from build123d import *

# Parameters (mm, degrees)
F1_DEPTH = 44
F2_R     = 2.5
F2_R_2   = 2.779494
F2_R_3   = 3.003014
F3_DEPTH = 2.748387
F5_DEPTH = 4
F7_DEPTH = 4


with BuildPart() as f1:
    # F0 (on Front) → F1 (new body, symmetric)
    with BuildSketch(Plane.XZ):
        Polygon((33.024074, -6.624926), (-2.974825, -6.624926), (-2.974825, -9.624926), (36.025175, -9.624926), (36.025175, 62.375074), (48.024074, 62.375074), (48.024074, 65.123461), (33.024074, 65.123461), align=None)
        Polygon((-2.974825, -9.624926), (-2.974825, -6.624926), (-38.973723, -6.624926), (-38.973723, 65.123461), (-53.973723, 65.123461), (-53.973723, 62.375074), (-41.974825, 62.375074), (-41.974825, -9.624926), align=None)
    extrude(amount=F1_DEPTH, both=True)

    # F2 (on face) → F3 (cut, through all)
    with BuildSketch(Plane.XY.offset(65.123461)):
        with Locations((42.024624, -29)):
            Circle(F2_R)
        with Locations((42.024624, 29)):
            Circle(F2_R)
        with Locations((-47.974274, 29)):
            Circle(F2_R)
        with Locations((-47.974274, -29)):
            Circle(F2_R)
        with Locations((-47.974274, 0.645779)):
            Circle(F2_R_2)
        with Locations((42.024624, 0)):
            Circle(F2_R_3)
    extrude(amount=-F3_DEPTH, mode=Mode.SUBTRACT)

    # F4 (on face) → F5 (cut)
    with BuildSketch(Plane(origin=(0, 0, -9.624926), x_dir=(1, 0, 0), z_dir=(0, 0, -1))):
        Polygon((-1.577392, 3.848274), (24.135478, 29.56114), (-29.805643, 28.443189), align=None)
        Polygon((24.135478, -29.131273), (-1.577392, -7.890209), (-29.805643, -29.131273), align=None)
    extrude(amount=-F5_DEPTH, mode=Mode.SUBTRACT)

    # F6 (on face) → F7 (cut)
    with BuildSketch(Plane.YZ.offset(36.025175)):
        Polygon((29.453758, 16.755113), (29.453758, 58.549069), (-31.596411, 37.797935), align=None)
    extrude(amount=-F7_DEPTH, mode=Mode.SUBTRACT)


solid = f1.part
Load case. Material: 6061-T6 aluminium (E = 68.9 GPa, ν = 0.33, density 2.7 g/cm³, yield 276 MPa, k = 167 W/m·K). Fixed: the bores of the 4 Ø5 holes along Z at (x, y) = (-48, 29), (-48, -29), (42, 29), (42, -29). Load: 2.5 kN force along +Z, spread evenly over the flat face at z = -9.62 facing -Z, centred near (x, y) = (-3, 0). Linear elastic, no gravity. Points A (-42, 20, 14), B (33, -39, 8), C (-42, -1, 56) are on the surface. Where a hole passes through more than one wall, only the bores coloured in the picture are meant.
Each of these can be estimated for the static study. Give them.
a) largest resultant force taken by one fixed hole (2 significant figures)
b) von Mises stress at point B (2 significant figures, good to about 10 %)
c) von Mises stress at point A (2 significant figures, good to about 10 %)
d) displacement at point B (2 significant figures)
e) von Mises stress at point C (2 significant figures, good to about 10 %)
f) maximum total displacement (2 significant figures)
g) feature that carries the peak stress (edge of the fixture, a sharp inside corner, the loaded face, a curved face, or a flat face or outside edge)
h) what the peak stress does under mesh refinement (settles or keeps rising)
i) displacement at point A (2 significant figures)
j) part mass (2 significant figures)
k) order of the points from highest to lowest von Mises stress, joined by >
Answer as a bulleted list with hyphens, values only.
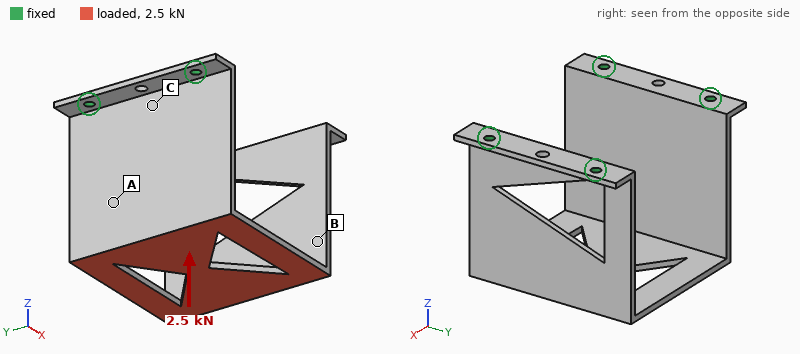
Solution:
- 680 N
- 71 MPa
- 39 MPa
- 0.24 mm
- 12 MPa
- 0.59 mm
- a sharp inside corner
- keeps rising
- 0.094 mm
- 150 g
- B > A > C
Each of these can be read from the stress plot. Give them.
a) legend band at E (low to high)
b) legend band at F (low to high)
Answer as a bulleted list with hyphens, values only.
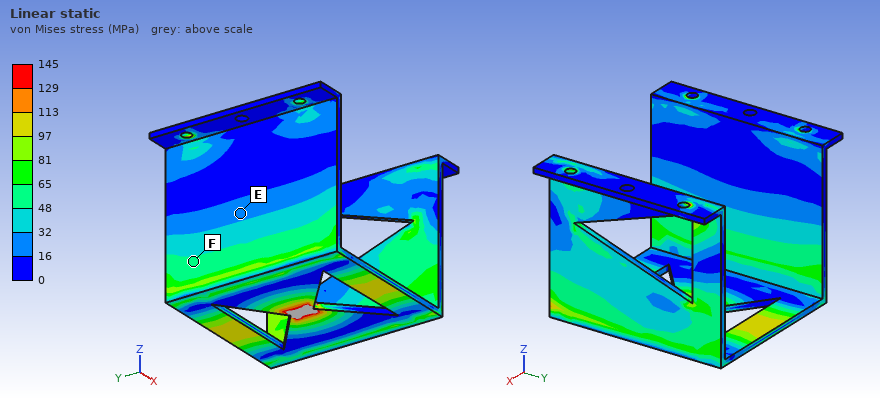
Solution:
- 16 to 32 MPa
- 48 to 65 MPa
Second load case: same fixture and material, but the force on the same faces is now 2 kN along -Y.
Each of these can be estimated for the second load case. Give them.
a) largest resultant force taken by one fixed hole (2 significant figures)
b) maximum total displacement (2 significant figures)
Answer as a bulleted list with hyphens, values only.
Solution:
- 1.4 kN
- 0.23 mm
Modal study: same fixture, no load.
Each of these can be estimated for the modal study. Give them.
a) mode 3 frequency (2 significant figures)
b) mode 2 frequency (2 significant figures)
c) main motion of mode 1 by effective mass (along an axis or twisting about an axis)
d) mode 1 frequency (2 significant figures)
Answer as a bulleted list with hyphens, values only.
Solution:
- 1500 Hz
- 1500 Hz
- along X
- 370 Hz
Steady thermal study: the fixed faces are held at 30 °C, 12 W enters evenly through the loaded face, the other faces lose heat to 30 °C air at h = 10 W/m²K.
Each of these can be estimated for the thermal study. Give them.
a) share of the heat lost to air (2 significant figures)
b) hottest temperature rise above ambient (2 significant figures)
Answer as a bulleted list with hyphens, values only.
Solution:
- 23 %
- 16 K
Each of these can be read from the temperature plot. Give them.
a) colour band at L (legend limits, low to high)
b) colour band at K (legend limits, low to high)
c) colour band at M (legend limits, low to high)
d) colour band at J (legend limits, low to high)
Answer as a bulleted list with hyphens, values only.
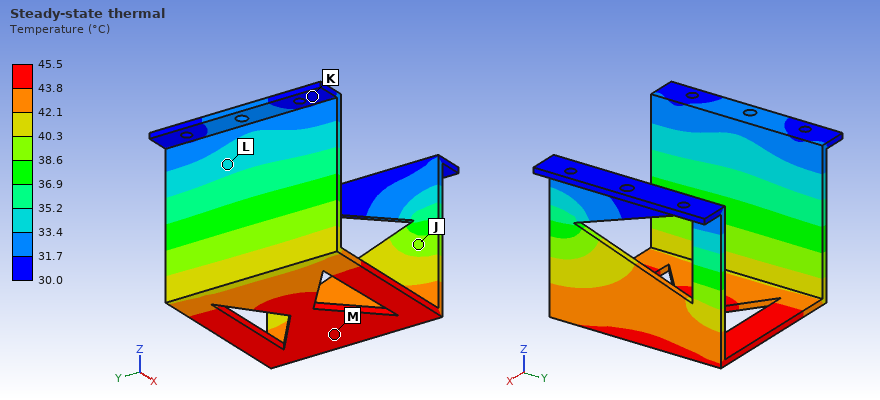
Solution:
- 33.4 to 35.2 °C
- 30.0 to 31.7 °C
- 43.8 to 45.5 °C
- 38.6 to 40.3 °C
